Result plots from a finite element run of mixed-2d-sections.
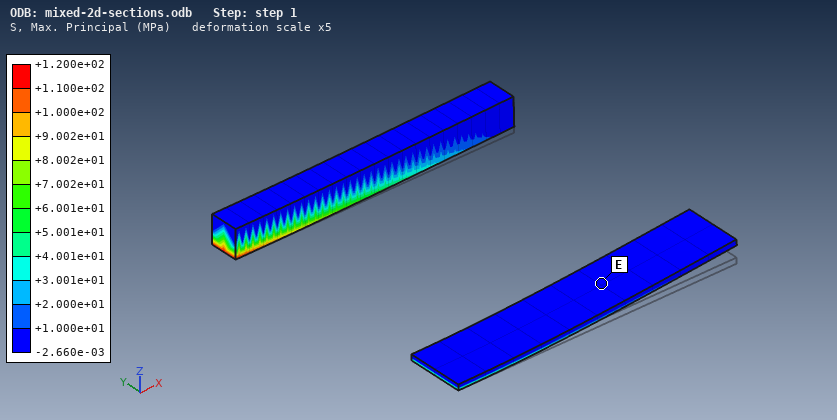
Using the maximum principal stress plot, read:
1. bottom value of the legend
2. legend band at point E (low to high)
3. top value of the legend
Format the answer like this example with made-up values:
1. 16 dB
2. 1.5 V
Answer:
1. -2.660e-03 MPa
2. -2.660e-03 to +1.000e+01 MPa
3. +1.200e+02 MPa
